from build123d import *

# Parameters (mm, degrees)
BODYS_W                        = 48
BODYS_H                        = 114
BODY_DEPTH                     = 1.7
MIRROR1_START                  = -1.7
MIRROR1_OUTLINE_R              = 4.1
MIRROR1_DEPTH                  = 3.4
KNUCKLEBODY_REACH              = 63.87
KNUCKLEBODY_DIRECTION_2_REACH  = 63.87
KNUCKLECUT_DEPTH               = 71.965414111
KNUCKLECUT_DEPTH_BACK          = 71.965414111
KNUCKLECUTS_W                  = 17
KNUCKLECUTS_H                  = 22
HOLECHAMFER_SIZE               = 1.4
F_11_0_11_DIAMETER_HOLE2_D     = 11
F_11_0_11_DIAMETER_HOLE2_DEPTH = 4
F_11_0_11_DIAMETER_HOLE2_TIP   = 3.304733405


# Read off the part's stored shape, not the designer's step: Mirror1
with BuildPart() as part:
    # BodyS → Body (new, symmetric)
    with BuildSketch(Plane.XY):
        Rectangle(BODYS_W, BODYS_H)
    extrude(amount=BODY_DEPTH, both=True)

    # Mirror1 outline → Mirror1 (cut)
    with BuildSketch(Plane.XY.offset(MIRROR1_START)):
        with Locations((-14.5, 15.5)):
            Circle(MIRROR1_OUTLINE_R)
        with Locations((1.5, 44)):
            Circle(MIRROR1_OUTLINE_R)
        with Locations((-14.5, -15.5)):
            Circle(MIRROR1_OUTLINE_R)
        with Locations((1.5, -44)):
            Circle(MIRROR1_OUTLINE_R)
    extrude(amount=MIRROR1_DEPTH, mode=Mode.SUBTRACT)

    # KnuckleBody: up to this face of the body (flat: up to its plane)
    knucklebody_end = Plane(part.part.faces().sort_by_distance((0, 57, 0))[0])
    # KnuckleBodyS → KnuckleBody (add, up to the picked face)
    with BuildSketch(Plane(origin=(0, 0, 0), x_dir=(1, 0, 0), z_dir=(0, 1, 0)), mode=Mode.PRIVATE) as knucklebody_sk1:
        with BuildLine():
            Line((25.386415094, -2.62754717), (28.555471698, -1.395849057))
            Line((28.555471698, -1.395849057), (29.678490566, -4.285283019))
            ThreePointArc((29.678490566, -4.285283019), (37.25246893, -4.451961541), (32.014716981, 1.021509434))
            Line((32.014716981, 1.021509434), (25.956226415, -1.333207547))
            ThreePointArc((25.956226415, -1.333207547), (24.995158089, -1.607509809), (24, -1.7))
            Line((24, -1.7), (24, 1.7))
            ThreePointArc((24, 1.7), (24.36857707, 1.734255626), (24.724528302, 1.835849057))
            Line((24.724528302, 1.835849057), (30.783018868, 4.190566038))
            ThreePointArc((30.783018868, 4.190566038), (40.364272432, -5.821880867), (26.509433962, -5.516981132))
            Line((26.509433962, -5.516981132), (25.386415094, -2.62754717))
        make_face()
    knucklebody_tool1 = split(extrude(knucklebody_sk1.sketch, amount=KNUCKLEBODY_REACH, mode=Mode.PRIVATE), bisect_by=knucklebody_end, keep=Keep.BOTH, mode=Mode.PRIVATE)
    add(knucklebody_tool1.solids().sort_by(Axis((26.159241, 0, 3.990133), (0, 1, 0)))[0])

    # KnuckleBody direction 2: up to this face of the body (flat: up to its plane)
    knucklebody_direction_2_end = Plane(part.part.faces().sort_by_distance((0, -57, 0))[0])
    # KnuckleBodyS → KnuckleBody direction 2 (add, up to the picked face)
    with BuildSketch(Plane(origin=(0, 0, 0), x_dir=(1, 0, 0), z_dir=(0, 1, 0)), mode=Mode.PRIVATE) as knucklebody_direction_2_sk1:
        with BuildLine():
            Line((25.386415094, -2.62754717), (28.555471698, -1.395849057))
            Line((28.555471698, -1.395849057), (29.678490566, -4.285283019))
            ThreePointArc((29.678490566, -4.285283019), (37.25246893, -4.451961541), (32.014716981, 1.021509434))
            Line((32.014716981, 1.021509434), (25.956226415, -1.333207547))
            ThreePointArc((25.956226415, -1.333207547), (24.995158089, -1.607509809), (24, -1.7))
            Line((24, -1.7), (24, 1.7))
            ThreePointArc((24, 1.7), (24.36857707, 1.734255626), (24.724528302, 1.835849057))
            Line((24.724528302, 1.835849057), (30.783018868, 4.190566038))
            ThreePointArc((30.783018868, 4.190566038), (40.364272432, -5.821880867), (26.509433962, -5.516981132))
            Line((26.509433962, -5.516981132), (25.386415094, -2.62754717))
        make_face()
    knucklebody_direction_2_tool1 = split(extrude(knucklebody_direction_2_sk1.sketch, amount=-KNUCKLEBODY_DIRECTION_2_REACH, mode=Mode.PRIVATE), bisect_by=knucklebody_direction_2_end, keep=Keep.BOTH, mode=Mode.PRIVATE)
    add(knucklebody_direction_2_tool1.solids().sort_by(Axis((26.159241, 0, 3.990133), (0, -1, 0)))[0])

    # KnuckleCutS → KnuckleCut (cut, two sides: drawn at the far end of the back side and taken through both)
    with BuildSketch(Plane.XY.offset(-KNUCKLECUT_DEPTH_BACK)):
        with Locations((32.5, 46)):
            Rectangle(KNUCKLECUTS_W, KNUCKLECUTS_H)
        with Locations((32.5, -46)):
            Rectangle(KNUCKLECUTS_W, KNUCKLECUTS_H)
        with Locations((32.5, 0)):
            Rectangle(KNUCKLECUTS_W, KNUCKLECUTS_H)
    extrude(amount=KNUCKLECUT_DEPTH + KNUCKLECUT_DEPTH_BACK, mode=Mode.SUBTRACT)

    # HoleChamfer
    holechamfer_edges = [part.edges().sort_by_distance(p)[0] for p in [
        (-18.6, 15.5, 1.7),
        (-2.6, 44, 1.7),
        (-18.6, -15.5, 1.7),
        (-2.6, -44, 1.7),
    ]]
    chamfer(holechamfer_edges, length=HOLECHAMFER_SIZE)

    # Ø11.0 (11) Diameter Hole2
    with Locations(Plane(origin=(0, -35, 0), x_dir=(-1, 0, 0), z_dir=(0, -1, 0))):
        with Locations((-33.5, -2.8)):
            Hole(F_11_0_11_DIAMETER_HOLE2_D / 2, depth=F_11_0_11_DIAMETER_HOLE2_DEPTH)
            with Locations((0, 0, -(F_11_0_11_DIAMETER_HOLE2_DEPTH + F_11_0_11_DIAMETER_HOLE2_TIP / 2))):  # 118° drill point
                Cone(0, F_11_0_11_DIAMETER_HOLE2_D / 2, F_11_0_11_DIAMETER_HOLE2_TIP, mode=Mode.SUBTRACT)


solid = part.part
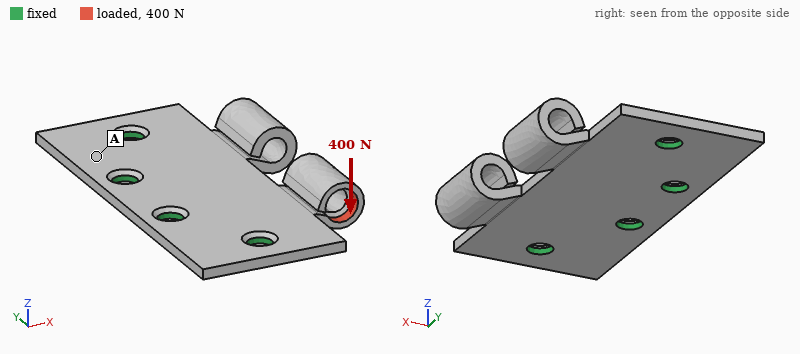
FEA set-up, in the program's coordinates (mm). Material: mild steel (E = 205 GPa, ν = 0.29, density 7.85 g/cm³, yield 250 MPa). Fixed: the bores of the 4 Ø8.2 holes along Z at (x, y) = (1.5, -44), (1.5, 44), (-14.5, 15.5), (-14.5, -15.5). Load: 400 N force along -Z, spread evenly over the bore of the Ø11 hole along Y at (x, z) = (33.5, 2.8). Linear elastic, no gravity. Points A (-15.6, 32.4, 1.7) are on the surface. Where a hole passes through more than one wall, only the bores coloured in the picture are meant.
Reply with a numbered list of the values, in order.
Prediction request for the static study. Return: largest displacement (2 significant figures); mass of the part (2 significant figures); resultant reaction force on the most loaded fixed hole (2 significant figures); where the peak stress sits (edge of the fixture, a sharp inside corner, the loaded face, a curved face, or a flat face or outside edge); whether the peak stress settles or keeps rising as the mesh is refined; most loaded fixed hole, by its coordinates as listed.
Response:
1. 0.26 mm
2. 190 g
3. 420 N
4. edge of the fixture
5. keeps rising
6. (1.5, -44)
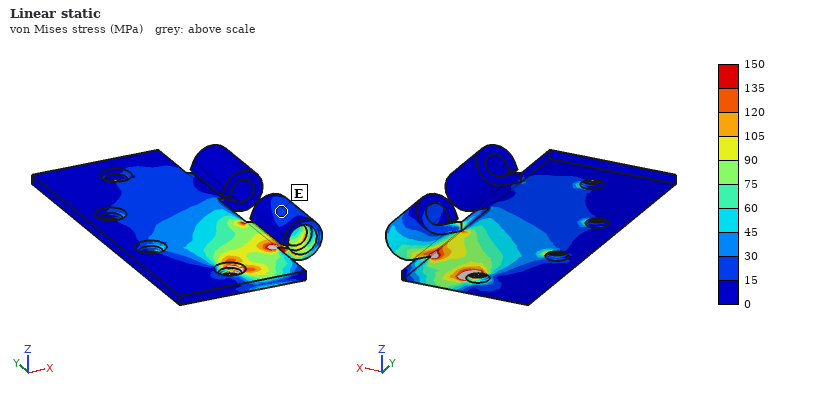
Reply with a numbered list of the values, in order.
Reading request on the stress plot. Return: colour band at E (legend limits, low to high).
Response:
1. 15 to 30 MPa
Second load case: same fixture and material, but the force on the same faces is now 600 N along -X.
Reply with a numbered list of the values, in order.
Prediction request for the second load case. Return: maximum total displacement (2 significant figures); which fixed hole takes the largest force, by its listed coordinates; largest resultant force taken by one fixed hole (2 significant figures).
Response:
1. 88 µm
2. (1.5, -44)
3. 380 N
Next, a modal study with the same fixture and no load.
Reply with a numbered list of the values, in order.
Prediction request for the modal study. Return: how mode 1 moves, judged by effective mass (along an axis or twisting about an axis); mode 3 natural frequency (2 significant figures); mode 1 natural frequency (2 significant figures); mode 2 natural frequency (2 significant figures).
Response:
1. along Z
2. 3400 Hz
3. 1200 Hz
4. 1700 Hz
